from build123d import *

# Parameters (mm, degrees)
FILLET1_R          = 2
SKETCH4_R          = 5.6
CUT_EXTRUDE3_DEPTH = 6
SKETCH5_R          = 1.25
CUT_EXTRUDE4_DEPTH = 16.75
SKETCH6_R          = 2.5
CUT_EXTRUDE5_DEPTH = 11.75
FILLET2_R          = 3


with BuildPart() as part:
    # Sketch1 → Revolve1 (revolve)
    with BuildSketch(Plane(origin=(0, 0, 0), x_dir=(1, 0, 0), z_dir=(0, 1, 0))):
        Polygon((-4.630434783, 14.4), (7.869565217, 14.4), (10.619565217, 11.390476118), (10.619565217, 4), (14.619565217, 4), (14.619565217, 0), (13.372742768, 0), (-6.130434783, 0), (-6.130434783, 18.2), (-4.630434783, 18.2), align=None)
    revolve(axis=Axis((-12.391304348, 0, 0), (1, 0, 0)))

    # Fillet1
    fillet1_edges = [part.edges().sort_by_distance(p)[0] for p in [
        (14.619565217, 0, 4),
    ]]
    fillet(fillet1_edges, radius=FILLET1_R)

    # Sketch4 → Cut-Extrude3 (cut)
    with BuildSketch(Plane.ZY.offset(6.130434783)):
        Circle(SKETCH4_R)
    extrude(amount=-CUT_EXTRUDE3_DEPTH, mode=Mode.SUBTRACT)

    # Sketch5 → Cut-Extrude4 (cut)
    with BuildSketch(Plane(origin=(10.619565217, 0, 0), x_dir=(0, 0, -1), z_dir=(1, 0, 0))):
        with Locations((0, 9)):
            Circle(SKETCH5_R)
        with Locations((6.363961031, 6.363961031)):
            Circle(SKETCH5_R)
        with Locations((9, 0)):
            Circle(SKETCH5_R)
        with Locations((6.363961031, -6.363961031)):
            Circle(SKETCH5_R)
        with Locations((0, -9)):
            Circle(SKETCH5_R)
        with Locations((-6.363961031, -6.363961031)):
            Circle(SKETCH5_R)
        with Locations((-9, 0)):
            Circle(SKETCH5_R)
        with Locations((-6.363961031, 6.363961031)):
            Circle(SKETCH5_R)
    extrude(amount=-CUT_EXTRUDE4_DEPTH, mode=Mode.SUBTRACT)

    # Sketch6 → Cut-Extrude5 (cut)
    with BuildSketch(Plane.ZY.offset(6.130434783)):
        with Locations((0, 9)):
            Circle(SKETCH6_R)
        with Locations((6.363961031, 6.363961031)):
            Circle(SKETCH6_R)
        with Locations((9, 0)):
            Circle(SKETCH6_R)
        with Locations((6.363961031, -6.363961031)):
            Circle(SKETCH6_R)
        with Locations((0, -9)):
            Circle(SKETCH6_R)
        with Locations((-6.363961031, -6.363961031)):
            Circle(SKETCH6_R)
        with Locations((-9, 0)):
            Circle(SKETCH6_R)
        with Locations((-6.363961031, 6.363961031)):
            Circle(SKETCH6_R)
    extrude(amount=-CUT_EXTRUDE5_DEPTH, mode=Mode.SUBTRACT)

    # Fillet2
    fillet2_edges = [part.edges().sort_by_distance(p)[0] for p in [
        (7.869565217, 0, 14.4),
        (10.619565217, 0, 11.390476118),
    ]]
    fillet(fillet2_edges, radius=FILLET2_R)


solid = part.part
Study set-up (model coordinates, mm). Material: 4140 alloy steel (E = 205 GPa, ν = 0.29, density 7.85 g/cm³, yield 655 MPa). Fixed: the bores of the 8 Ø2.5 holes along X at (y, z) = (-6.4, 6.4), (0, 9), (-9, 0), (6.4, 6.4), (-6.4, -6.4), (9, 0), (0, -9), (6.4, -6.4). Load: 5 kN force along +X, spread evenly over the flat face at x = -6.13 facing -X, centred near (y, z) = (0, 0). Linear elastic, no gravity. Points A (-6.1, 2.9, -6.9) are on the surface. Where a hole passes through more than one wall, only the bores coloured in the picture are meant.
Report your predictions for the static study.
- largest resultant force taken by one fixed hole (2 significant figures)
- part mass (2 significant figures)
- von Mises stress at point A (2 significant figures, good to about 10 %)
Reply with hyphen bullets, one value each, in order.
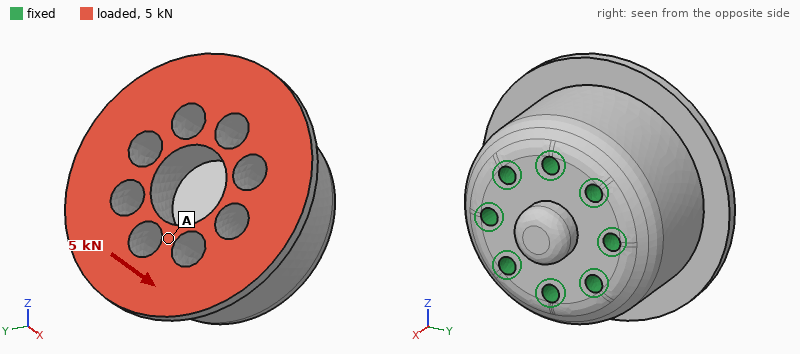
- 630 N
- 68 g
- 16 MPa
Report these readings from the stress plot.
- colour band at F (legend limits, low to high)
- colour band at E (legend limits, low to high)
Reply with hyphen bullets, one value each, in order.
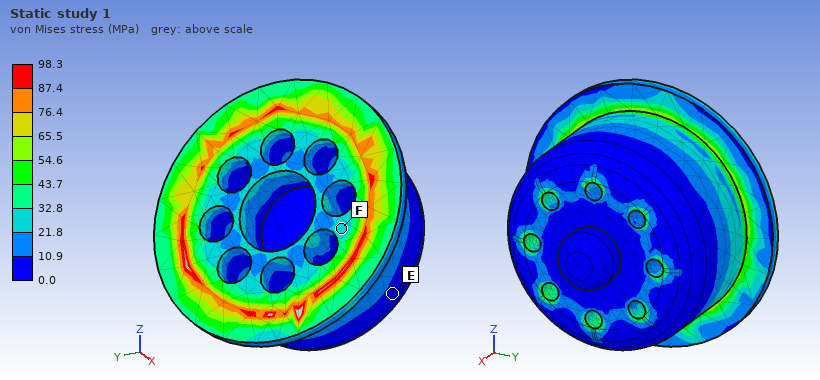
- 21.8 to 32.8 MPa
- 0.0 to 10.9 MPa
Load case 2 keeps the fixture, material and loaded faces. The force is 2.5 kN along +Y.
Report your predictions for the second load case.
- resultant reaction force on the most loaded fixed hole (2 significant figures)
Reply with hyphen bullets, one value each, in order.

- 810 N
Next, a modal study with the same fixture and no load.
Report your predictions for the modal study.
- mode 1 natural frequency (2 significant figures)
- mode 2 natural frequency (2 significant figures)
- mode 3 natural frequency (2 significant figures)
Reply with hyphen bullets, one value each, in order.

- 30 kHz
- 30 kHz
- 39 kHz
